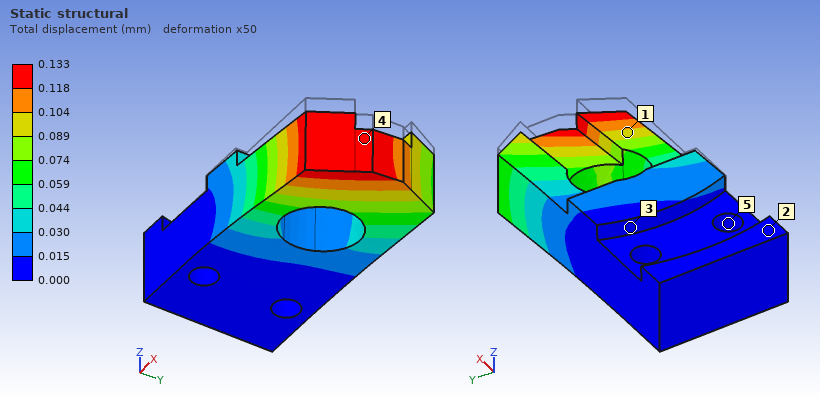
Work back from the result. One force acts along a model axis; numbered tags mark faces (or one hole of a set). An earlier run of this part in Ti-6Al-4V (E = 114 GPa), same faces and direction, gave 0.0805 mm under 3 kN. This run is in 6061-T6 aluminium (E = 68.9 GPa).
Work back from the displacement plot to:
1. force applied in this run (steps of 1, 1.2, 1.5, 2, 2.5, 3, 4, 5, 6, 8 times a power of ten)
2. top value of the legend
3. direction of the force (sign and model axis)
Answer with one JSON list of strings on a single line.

["3 kN", "0.133 mm", "-Z"]
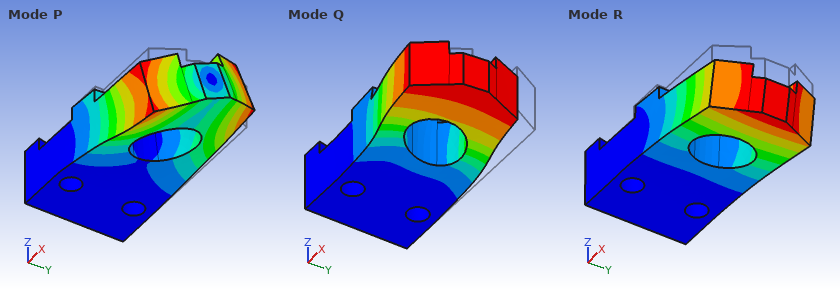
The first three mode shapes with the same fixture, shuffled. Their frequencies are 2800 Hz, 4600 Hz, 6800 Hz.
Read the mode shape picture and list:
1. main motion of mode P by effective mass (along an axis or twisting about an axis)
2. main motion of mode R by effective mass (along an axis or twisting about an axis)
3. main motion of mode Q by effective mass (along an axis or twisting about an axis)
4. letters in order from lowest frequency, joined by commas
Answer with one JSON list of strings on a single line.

["twisting about X", "along Z", "along Y", "R, Q, P"]
